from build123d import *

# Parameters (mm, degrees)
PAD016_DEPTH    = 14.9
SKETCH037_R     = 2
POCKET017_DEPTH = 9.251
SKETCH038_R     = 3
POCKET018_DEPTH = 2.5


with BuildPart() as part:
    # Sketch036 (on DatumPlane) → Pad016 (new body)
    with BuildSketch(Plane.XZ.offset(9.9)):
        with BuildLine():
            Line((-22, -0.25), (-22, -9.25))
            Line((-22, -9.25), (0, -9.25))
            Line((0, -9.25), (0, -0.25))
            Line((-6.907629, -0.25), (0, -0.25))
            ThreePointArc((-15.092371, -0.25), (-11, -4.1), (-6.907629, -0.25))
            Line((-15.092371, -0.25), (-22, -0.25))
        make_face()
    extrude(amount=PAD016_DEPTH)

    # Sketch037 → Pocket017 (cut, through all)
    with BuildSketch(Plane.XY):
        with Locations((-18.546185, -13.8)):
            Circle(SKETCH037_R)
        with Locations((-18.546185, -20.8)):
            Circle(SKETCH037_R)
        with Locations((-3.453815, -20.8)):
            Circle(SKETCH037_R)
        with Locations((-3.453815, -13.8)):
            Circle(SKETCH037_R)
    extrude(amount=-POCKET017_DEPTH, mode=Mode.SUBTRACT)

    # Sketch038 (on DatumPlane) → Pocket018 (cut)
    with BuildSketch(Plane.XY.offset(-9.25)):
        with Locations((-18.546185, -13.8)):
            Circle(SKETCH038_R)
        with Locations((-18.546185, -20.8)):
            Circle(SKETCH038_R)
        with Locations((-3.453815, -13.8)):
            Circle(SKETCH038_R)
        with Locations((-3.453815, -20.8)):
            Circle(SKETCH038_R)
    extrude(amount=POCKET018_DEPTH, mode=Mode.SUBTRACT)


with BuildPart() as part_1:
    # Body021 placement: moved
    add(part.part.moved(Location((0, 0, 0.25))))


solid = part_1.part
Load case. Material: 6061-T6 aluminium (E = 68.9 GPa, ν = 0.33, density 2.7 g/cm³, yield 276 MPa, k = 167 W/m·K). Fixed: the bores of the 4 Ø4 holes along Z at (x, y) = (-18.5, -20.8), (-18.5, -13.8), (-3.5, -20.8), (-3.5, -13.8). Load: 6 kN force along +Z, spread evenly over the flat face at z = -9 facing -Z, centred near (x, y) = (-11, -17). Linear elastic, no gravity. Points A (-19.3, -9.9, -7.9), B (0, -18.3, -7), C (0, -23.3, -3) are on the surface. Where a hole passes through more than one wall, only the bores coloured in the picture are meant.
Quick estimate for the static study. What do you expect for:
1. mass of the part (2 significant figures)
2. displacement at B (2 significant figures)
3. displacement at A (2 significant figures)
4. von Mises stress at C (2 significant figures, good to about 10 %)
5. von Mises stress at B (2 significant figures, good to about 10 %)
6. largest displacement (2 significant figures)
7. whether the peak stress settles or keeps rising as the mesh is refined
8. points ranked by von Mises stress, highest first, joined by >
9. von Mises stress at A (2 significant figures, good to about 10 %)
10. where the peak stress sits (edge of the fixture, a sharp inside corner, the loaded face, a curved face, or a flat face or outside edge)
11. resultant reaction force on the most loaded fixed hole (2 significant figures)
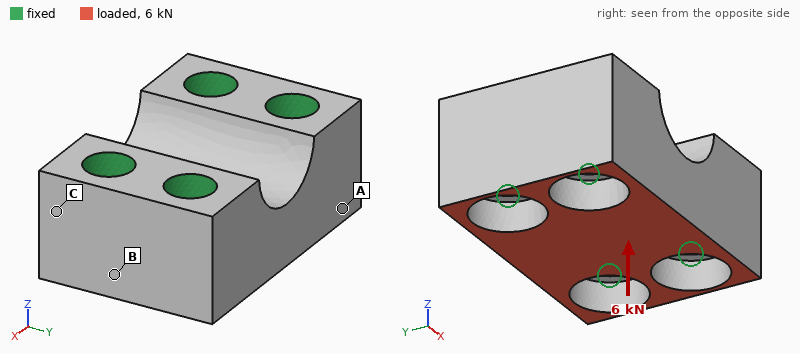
5.3 g
1.2 µm
2.4 µm
9.6 MPa
18 MPa
6.6 µm
keeps rising
A > B > C
28 MPa
edge of the fixture
1.6 kN
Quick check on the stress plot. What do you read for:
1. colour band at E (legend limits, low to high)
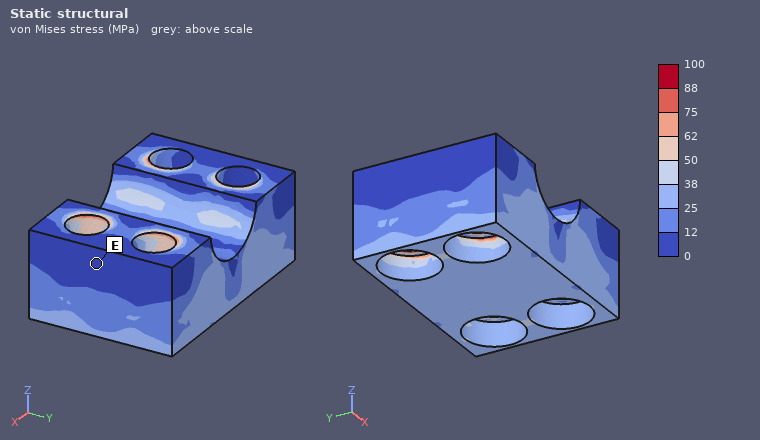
0 to 12 MPa
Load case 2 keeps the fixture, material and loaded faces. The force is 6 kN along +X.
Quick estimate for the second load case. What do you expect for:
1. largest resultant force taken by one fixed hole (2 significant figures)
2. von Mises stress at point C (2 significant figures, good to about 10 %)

1.7 kN
22 MPa
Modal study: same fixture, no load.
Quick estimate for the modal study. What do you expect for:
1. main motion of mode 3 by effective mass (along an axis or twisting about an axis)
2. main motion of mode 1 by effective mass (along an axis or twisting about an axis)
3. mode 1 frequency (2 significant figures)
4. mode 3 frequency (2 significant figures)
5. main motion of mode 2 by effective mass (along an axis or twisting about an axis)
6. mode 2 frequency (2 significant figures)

along Y
along Y
88 kHz
120 kHz
along Z
100 kHz
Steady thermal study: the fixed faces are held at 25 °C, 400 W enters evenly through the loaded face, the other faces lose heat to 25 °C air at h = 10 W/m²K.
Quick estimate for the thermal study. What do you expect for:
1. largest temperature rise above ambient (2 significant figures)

76 K
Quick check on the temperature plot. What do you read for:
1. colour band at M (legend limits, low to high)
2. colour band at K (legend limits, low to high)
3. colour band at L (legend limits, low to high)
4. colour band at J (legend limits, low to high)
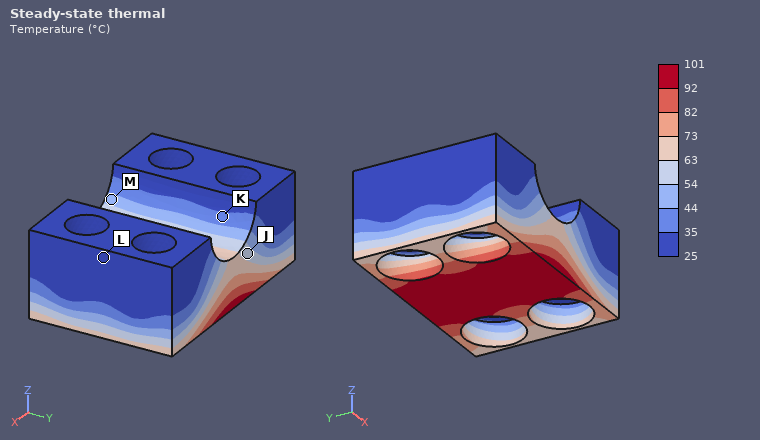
44 to 54 °C
35 to 44 °C
25 to 35 °C
54 to 63 °C
